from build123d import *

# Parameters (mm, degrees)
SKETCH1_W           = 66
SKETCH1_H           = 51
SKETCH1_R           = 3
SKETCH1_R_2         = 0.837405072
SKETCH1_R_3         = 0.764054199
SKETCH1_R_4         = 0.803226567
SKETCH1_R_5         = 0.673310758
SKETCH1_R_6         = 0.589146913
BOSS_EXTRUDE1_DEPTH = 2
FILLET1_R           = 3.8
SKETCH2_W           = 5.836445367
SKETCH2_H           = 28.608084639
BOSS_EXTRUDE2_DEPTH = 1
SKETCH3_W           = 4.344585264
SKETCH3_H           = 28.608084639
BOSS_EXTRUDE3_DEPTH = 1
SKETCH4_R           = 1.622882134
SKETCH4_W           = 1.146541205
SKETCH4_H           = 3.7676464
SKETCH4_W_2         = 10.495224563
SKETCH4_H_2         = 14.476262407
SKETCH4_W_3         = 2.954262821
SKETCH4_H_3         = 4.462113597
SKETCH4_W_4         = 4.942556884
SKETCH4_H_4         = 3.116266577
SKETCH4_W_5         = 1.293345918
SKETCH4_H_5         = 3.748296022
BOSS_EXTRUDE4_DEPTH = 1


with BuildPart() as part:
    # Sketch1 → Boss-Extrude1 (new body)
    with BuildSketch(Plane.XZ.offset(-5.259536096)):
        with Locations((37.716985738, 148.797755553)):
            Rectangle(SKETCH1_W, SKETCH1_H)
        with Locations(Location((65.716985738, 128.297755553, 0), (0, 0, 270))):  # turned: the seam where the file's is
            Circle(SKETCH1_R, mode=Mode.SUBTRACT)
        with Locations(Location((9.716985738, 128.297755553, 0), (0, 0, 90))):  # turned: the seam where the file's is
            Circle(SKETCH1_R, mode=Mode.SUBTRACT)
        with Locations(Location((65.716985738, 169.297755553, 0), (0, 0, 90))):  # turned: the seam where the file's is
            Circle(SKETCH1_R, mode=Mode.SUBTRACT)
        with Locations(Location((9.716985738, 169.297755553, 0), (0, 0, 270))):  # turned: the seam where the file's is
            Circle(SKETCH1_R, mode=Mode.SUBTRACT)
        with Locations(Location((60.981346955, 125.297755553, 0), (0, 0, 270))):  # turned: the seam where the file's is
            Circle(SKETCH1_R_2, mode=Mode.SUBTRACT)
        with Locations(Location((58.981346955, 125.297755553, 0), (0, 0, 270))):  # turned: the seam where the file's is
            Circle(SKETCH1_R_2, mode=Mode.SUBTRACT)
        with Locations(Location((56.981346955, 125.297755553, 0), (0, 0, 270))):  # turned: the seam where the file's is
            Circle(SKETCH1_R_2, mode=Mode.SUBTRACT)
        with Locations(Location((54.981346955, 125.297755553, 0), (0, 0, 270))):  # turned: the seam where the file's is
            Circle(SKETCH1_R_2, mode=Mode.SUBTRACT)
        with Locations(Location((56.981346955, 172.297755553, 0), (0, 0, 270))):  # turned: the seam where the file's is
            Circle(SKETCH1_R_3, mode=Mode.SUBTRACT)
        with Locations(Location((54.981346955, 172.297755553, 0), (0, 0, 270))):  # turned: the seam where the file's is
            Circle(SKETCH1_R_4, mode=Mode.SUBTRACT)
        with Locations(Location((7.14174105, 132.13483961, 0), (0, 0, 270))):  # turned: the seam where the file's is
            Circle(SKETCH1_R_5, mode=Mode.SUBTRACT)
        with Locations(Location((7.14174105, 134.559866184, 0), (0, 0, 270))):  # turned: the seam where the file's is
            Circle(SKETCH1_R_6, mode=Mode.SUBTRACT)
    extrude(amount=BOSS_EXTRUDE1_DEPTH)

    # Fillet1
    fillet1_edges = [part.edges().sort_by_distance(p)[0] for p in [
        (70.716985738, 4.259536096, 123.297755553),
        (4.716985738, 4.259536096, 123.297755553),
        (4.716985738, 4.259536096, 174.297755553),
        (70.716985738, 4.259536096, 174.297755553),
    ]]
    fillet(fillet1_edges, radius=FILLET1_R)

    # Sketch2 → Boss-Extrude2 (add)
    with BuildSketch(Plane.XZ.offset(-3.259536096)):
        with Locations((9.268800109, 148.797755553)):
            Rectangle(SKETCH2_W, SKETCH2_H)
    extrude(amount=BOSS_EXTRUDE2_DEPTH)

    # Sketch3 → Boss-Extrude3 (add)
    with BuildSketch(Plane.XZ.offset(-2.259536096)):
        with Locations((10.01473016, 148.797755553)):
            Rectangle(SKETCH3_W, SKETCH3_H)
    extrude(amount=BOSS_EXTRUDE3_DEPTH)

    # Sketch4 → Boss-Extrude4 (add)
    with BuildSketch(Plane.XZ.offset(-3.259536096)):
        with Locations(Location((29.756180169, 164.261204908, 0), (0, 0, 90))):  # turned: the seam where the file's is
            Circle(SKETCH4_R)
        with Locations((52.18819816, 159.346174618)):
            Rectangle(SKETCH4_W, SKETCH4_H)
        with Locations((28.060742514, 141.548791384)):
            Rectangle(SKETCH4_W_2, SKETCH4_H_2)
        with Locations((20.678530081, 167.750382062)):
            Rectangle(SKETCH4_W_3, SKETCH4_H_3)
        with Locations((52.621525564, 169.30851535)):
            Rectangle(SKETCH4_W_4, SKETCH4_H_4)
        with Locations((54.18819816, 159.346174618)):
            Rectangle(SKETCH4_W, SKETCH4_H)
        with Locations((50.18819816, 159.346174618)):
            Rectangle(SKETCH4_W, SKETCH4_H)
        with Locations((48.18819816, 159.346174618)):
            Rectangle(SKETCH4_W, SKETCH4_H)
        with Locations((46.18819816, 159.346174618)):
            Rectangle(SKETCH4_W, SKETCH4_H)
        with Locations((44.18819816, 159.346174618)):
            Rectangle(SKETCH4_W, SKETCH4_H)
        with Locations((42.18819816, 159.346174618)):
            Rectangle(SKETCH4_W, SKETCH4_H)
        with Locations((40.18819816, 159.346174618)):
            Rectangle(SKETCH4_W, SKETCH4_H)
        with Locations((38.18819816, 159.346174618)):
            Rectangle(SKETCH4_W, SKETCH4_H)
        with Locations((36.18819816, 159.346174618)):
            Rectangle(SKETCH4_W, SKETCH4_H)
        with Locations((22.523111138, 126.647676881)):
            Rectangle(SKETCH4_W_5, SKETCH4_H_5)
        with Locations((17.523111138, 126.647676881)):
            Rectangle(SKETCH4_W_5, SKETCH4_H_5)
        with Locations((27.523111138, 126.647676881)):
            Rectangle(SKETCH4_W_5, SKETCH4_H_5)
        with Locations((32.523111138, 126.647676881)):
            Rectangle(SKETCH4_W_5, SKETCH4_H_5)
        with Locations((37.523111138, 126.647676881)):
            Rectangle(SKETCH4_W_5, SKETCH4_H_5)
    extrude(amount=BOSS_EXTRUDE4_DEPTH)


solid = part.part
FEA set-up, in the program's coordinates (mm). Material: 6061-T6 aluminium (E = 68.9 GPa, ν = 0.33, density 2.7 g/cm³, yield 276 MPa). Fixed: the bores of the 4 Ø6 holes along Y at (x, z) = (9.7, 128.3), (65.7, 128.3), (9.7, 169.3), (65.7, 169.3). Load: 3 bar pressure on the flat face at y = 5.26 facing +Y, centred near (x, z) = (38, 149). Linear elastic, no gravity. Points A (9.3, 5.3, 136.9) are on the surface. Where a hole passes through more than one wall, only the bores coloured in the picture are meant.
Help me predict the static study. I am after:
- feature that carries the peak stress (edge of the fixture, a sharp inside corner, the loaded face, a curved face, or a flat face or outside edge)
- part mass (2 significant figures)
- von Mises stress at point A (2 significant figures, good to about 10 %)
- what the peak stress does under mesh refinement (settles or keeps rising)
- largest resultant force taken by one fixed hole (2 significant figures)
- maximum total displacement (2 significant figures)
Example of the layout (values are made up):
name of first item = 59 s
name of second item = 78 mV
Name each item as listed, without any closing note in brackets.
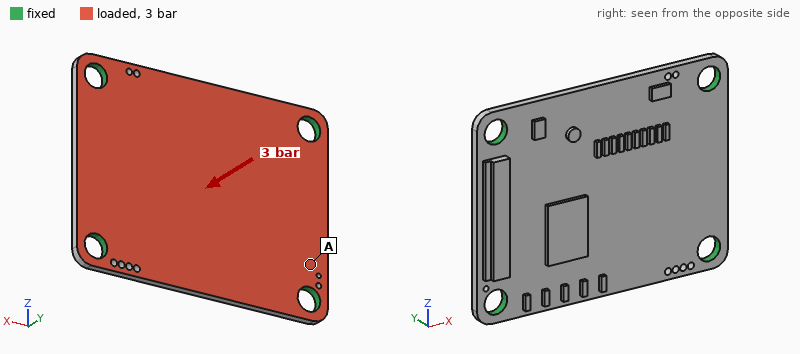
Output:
feature that carries the peak stress = a sharp inside corner
part mass = 19 g
von Mises stress at point A = 31 MPa
what the peak stress does under mesh refinement = keeps rising
largest resultant force taken by one fixed hole = 270 N
maximum total displacement = 0.18 mm
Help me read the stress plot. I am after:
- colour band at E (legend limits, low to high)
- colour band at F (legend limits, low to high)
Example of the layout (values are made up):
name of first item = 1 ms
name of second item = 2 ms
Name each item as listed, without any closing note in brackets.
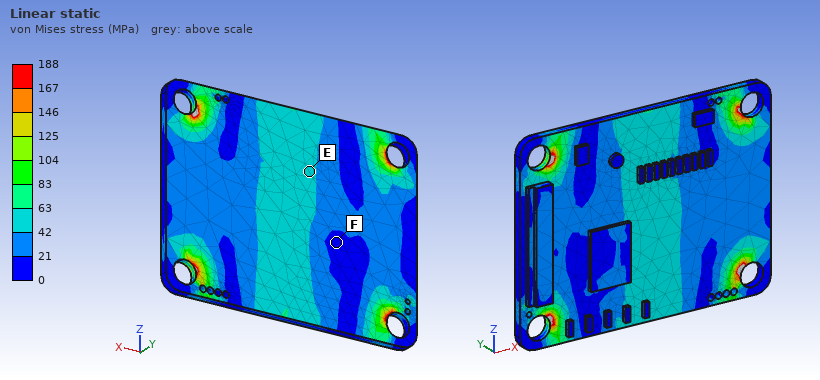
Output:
colour band at E = 42 to 63 MPa
colour band at F = 0 to 21 MPa
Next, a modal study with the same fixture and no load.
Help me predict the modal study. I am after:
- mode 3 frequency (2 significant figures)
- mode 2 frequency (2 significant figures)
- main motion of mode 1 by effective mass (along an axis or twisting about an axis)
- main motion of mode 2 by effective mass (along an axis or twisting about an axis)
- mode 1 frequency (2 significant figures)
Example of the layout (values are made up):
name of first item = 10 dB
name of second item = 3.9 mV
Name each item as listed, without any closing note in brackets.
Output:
mode 3 frequency = 6800 Hz
mode 2 frequency = 4700 Hz
main motion of mode 1 by effective mass = along Y
main motion of mode 2 by effective mass = twisting about X
mode 1 frequency = 3200 Hz
